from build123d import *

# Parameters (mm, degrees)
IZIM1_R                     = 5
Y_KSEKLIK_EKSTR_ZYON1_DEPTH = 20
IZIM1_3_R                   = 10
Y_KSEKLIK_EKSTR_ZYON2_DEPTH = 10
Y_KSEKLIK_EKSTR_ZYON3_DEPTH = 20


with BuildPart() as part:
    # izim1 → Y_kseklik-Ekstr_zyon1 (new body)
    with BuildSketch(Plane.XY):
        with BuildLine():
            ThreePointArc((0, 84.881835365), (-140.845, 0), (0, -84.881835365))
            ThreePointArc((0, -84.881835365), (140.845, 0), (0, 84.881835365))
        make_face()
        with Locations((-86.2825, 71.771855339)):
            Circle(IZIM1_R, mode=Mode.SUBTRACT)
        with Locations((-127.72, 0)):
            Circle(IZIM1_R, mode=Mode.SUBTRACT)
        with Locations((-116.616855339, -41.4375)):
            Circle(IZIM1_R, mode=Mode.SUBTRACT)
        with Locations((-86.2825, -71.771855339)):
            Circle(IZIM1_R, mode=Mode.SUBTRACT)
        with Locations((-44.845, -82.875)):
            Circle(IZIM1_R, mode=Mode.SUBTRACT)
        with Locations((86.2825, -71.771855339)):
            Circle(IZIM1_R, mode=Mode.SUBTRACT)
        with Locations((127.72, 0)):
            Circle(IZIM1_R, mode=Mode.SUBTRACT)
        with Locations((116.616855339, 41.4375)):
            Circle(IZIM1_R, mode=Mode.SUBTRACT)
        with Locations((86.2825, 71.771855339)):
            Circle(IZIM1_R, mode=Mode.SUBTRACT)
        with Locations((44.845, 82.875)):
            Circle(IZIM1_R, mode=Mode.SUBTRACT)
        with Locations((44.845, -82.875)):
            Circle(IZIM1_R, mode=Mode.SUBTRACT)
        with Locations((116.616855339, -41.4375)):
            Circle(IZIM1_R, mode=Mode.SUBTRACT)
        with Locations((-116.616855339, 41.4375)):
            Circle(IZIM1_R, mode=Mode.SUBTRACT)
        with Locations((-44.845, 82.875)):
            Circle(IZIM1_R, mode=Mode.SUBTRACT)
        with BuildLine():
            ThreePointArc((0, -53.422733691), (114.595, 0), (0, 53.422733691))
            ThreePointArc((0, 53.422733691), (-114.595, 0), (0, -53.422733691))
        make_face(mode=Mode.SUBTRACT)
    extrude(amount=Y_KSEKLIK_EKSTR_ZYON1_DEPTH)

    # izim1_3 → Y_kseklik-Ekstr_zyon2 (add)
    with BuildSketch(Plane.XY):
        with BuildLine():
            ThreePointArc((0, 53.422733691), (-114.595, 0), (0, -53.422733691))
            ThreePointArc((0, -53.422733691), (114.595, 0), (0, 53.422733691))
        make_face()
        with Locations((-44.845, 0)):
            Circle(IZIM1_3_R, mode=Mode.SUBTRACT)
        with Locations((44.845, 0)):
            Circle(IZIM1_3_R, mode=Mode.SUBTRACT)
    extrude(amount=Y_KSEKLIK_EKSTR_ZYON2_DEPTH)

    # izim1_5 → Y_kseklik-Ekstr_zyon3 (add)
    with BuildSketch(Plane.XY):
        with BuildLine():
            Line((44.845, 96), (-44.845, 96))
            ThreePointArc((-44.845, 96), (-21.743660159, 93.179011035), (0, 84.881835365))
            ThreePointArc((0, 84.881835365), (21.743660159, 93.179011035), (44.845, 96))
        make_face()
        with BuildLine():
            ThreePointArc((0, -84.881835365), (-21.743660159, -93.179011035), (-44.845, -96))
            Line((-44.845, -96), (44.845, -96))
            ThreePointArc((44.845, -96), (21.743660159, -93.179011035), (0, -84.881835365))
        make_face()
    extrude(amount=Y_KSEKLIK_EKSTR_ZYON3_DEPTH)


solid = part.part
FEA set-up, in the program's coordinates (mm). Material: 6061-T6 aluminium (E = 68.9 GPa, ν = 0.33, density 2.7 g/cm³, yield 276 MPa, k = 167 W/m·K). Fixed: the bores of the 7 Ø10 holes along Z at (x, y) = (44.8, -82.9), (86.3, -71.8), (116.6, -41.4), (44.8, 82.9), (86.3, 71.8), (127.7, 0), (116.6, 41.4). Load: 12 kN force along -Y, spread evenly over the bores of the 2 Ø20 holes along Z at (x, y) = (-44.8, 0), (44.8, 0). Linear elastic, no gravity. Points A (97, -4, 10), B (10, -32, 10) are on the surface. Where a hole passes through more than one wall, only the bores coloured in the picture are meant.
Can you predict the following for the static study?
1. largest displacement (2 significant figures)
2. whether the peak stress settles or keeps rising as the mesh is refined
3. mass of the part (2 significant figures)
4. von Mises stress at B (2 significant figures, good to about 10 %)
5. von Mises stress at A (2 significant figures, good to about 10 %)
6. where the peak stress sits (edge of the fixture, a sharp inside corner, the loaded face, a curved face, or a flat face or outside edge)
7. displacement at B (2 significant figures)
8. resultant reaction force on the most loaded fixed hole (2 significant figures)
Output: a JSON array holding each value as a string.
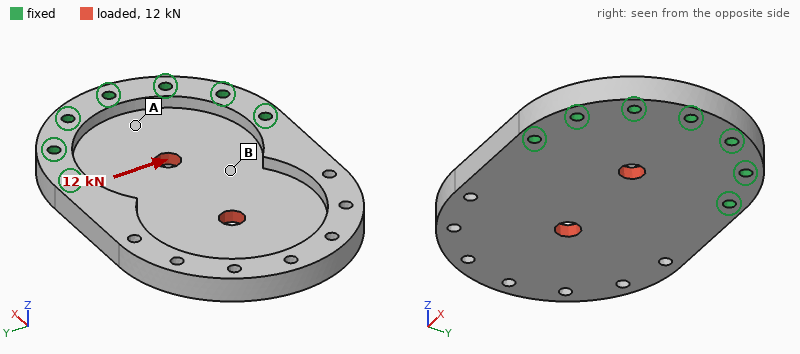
["24 µm", "keeps rising", "1.7 kg", "6.7 MPa", "2.1 MPa", "edge of the fixture", "10.0 µm", "5.2 kN"]
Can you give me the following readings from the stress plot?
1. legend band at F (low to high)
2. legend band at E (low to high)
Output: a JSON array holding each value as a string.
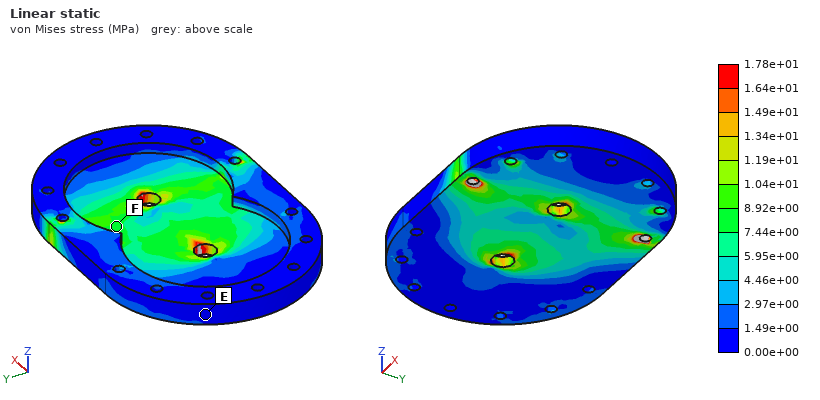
["7.44e+00 to 8.92e+00 MPa", "0.00e+00 to 1.49e+00 MPa"]
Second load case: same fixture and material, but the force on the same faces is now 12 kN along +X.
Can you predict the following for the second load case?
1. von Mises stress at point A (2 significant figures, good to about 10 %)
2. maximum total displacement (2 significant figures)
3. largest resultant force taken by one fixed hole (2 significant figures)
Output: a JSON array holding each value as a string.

["5.8 MPa", "61 µm", "2.5 kN"]
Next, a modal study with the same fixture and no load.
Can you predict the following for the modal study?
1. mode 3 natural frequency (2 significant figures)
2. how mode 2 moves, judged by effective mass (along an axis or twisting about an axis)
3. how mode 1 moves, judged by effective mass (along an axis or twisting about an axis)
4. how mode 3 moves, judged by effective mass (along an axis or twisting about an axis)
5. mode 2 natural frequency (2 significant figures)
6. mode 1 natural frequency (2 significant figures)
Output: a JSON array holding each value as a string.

["2000 Hz", "twisting about X", "along Z", "along Z", "1100 Hz", "430 Hz"]
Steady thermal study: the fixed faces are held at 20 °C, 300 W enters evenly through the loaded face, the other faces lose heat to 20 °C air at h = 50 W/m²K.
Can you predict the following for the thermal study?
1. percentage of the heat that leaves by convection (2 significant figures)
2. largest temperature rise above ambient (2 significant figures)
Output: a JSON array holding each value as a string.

["34 %", "50 K"]
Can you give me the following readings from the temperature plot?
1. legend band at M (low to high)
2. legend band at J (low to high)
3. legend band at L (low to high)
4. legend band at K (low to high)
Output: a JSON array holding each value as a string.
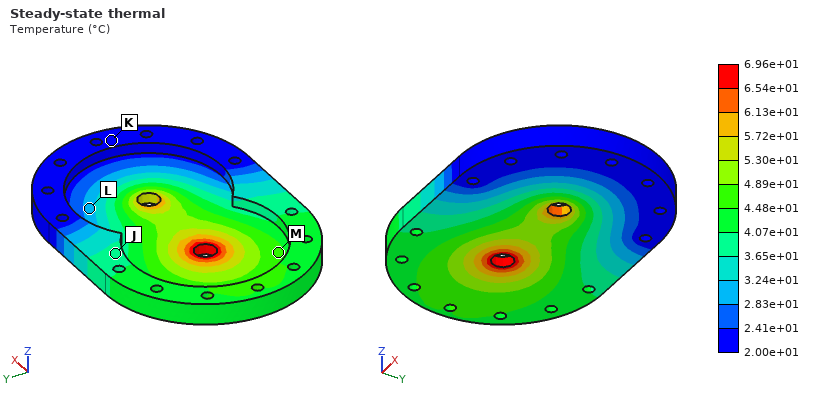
["4.48e+01 to 4.89e+01 °C", "3.65e+01 to 4.07e+01 °C", "2.83e+01 to 3.24e+01 °C", "2.00e+01 to 2.41e+01 °C"]
